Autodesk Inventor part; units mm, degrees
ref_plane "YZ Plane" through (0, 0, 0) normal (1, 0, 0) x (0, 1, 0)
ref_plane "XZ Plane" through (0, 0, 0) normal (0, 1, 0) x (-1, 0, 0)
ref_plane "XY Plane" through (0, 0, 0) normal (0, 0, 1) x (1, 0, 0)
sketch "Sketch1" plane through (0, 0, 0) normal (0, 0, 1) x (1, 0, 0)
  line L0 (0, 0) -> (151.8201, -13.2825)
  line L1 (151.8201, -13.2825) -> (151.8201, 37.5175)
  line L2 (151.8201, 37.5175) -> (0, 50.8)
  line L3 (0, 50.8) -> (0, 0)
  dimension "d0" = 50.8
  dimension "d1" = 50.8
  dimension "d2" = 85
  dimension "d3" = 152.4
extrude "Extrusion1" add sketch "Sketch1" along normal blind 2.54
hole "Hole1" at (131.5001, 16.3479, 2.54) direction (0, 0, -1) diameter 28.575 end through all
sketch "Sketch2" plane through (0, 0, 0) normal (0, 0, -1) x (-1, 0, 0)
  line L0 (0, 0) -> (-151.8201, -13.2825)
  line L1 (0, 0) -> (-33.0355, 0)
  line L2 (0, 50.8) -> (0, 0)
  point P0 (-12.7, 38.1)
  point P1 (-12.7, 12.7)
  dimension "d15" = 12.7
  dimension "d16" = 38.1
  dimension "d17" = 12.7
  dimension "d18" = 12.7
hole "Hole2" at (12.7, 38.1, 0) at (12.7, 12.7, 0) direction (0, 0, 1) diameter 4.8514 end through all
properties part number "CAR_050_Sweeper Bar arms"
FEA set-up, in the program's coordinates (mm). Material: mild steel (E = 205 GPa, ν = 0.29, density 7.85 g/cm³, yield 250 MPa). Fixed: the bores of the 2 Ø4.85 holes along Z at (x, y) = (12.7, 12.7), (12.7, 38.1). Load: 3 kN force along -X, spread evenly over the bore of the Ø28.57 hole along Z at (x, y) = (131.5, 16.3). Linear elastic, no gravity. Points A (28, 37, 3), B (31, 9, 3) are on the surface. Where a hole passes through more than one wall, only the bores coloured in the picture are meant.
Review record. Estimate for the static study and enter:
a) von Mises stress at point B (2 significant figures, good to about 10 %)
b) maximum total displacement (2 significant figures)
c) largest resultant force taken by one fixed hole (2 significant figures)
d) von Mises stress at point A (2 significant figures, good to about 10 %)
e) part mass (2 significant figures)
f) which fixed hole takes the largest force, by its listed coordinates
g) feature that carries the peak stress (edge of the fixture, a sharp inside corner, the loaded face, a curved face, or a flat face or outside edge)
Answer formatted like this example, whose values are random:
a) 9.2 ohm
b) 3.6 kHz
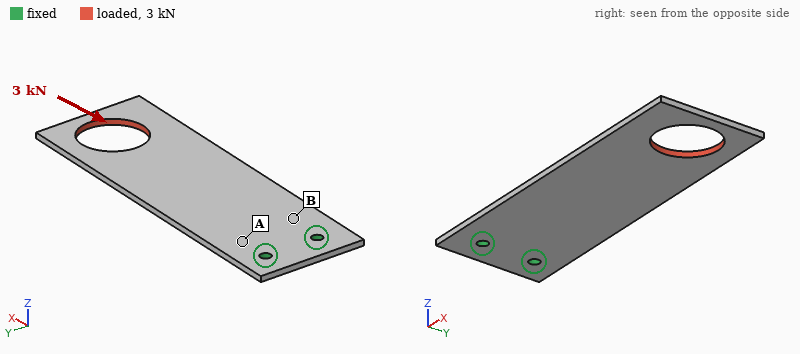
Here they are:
a) 36 MPa
b) 41 µm
c) 2.5 kN
d) 13 MPa
e) 140 g
f) (12.7, 12.7)
g) edge of the fixture
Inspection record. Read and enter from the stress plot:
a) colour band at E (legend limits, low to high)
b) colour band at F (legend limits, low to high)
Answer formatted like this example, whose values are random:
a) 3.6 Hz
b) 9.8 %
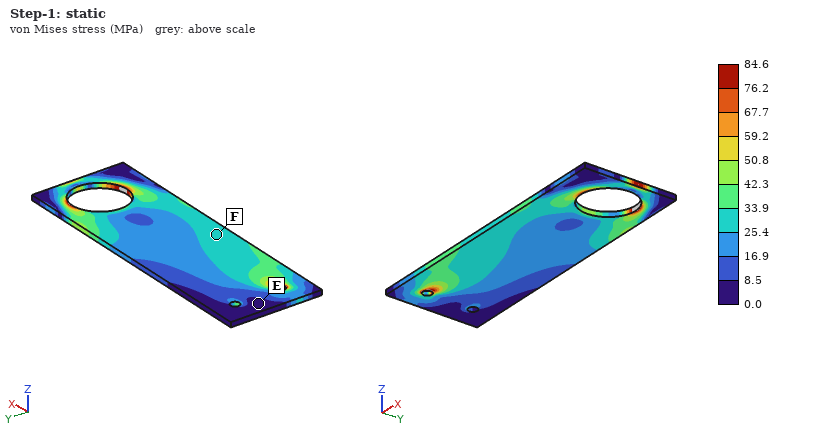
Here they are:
a) 0.0 to 8.5 MPa
b) 25.4 to 33.9 MPa
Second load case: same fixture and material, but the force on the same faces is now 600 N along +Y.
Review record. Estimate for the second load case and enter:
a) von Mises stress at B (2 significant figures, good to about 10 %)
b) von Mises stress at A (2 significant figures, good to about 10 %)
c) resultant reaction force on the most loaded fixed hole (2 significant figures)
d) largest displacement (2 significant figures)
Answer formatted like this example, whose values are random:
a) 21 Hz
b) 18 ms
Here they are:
a) 34 MPa
b) 42 MPa
c) 2.6 kN
d) 0.12 mm
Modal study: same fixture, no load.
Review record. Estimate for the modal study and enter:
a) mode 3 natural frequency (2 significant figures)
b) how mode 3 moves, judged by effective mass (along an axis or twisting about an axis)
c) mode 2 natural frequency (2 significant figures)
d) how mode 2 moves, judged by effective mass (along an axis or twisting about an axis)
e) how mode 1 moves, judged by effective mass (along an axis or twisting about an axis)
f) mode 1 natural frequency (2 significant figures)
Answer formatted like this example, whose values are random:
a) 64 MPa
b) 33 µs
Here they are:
a) 690 Hz
b) along Z
c) 610 Hz
d) twisting about X
e) along Z
f) 120 Hz
